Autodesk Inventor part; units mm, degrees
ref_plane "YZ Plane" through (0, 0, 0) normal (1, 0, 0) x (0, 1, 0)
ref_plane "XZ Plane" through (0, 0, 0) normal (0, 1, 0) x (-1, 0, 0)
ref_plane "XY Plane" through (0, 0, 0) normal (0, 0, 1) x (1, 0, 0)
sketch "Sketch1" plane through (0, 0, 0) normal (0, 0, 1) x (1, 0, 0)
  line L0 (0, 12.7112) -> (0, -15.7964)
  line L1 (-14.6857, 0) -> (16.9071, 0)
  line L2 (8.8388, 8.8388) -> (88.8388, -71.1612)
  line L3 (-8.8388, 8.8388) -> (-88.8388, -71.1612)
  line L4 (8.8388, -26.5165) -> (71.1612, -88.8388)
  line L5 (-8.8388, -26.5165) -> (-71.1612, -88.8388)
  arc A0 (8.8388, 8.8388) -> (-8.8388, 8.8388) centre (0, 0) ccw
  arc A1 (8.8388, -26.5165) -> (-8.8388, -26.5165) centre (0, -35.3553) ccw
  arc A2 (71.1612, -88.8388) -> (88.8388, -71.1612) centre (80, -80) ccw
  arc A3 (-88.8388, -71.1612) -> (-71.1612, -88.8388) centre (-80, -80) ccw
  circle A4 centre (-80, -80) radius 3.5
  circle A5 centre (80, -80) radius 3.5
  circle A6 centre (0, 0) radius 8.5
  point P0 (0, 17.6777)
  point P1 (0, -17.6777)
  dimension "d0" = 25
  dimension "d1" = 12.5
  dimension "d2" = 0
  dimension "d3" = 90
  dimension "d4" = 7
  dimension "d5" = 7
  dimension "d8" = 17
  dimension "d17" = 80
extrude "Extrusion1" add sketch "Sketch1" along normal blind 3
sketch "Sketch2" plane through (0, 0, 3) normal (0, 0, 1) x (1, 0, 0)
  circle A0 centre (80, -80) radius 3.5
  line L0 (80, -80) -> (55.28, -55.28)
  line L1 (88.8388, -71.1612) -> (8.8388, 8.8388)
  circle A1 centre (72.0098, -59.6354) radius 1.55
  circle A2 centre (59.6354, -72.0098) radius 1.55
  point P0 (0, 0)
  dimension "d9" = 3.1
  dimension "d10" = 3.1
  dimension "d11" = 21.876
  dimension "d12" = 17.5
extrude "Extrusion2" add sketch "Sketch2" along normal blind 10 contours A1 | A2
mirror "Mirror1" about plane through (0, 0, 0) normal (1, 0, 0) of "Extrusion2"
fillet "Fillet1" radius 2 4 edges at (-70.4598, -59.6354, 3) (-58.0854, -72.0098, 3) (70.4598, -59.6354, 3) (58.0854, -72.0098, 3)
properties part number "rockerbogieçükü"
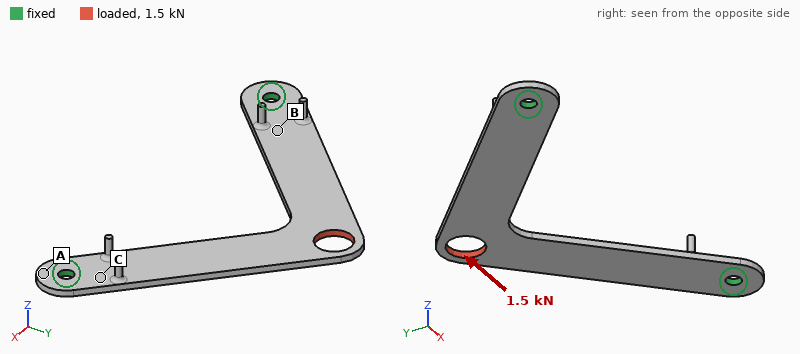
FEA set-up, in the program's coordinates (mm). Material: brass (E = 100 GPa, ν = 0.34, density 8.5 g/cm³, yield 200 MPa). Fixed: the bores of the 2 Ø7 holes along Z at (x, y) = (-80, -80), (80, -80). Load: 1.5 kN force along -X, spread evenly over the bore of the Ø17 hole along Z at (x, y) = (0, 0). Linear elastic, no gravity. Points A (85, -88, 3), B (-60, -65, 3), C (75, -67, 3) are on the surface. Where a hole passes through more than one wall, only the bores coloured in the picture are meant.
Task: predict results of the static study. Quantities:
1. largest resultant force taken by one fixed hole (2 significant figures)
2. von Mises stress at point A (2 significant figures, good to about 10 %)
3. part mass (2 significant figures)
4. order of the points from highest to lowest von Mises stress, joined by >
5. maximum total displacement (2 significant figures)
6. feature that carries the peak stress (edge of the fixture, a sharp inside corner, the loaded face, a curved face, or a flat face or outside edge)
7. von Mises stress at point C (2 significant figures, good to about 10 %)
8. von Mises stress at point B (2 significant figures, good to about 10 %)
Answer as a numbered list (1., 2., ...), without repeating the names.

1. 1.1 kN
2. 4.8 MPa
3. 150 g
4. C > B > A
5. 38 µm
6. the loaded face
7. 17 MPa
8. 13 MPa
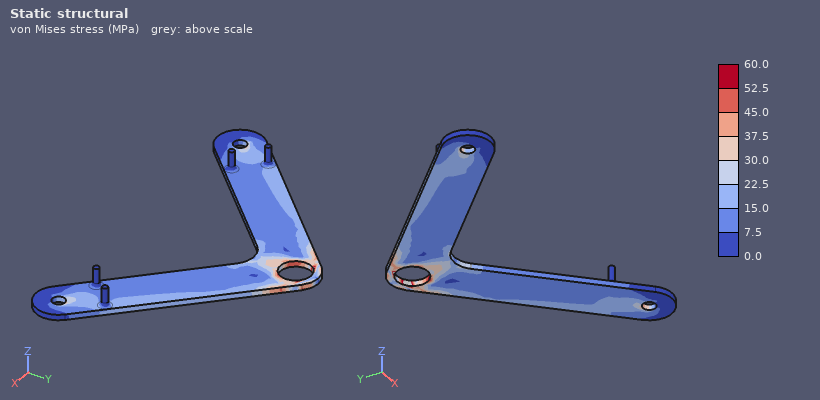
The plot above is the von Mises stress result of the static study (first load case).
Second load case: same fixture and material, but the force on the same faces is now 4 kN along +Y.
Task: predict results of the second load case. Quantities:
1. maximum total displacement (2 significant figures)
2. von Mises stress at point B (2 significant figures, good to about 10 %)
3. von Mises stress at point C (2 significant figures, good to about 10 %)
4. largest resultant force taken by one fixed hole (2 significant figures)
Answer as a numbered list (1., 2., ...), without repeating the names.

1. 68 µm
2. 39 MPa
3. 37 MPa
4. 2.8 kN
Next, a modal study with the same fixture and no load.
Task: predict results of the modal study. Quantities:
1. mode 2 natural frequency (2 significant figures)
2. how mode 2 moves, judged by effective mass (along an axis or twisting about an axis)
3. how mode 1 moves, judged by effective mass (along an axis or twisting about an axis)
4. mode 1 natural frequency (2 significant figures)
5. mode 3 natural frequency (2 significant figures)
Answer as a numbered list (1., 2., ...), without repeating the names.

1. 630 Hz
2. twisting about Y
3. along Z
4. 180 Hz
5. 890 Hz
